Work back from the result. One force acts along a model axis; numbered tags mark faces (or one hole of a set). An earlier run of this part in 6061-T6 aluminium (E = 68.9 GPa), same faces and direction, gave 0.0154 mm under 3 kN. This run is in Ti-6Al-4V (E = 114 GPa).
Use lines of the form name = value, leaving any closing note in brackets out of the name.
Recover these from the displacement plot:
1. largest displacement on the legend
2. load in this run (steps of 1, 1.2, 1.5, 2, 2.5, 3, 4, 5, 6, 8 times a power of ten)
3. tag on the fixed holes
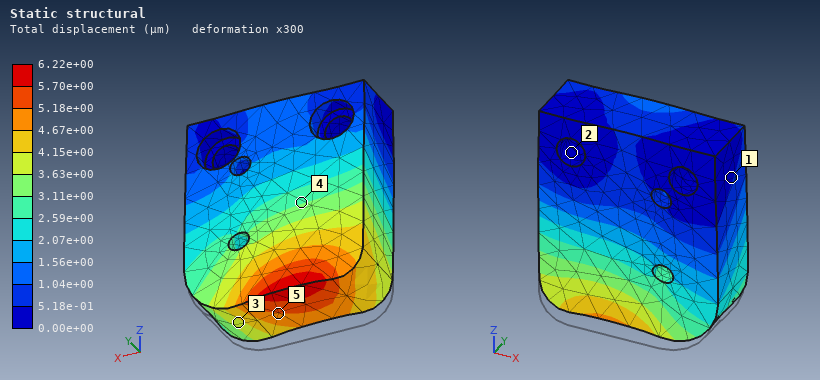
largest displacement on the legend = 6.22e+00 µm
load in this run = 2 kN
tag on the fixed holes = 2
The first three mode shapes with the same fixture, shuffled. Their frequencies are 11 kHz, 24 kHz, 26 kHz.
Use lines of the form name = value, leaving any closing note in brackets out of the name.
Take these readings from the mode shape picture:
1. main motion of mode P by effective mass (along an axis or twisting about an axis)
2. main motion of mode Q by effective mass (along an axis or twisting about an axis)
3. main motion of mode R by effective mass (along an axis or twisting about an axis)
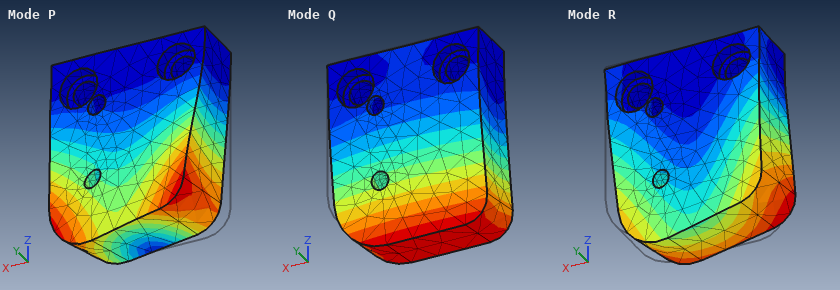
main motion of mode P by effective mass = along X
main motion of mode Q by effective mass = along Y
main motion of mode R by effective mass = along X
